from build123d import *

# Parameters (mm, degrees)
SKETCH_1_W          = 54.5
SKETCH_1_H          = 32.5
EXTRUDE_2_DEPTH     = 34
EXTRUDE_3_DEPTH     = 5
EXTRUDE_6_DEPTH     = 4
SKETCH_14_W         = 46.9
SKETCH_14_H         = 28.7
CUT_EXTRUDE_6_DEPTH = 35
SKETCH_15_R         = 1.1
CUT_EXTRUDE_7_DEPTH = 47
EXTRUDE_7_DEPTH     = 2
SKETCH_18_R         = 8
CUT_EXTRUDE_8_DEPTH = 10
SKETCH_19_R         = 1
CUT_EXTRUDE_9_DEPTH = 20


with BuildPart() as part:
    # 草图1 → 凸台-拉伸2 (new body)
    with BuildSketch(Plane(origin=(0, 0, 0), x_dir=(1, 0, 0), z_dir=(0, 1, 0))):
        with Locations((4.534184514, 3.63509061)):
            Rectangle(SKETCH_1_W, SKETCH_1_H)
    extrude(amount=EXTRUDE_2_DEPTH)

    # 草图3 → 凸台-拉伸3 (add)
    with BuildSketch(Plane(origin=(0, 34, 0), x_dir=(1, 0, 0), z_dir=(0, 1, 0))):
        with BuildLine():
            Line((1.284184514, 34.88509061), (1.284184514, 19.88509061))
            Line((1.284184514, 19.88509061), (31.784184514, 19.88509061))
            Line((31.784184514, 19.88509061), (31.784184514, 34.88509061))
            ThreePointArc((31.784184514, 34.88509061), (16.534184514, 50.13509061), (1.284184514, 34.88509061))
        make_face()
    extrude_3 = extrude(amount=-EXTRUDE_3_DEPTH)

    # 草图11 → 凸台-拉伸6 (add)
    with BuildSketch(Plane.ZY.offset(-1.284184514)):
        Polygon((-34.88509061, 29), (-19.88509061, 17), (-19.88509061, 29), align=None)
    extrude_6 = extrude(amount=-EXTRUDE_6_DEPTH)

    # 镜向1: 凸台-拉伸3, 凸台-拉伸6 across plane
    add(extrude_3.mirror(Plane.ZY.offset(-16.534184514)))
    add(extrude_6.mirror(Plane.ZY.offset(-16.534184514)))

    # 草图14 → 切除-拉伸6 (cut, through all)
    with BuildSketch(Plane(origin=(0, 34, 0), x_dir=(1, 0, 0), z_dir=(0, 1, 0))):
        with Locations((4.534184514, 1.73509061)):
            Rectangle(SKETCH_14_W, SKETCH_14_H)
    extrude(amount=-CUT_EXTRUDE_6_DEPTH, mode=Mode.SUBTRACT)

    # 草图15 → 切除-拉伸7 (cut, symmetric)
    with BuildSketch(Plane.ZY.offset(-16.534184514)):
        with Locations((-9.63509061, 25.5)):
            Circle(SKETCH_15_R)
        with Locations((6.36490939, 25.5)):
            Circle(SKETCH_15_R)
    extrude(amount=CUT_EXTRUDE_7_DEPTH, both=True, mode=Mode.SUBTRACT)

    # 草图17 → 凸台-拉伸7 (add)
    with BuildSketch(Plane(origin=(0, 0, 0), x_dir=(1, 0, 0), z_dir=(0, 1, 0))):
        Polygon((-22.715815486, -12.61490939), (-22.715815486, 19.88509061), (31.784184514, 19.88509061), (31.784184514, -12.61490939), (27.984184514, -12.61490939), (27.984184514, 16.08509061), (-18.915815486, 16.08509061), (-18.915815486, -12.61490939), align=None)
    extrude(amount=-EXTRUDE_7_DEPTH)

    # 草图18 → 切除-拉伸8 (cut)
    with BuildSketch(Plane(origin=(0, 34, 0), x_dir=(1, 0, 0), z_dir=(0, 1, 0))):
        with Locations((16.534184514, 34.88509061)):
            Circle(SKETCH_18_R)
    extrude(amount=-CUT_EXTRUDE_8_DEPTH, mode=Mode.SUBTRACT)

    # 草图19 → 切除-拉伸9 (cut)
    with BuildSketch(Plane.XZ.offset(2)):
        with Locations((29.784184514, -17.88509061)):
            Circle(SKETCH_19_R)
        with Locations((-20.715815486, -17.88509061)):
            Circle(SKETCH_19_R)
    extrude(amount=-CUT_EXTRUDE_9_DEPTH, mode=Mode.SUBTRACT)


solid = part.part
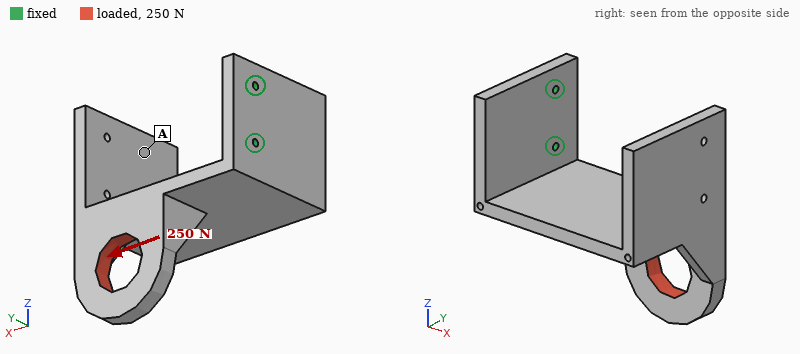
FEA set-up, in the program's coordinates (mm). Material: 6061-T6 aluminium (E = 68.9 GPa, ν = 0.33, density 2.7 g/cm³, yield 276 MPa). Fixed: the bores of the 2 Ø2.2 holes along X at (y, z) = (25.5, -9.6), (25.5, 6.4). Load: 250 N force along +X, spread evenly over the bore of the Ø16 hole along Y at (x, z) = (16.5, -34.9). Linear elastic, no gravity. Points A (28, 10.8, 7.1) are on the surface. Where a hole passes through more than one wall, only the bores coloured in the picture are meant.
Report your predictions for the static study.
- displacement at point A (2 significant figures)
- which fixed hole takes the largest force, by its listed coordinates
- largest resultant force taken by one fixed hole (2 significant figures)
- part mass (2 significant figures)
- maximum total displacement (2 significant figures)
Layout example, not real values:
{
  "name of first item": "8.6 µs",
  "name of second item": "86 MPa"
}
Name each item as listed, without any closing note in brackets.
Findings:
{
  "displacement at point A": "0.70 mm",
  "which fixed hole takes the largest force, by its listed coordinates": "(25.5, -9.6)",
  "largest resultant force taken by one fixed hole": "460 N",
  "part mass": "51 g",
  "maximum total displacement": "0.82 mm"
}
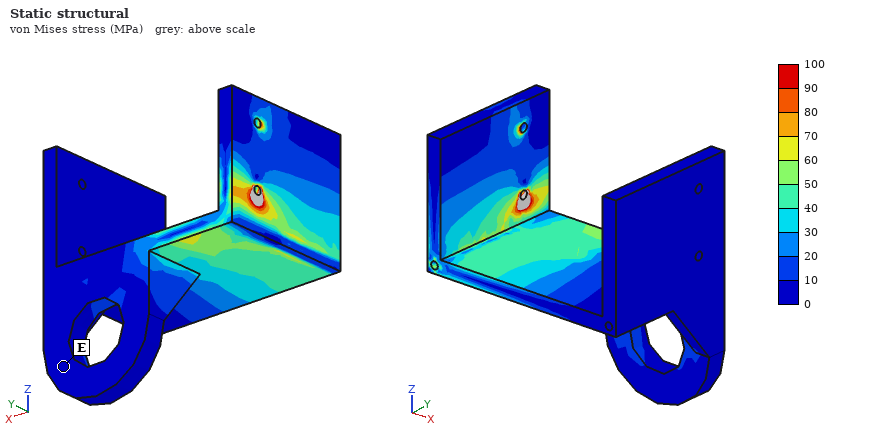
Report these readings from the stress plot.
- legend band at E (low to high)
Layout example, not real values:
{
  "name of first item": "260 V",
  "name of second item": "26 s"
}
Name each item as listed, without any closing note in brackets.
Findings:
{
  "legend band at E": "0 to 10 MPa"
}
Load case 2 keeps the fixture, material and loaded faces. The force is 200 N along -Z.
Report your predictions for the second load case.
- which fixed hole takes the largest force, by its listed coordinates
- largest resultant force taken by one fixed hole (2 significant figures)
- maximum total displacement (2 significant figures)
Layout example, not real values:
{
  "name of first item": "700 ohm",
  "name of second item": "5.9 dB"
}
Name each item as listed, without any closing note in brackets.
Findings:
{
  "which fixed hole takes the largest force, by its listed coordinates": "(25.5, -9.6)",
  "largest resultant force taken by one fixed hole": "320 N",
  "maximum total displacement": "1.1 mm"
}
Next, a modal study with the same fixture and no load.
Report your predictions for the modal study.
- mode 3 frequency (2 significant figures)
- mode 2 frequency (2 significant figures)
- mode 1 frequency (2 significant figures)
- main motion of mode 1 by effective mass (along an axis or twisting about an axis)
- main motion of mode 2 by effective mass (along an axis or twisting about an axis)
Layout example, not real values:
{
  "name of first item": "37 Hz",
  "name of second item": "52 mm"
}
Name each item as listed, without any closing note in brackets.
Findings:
{
  "mode 3 frequency": "1300 Hz",
  "mode 2 frequency": "660 Hz",
  "mode 1 frequency": "410 Hz",
  "main motion of mode 1 by effective mass": "along Z",
  "main motion of mode 2 by effective mass": "along Y"
}
